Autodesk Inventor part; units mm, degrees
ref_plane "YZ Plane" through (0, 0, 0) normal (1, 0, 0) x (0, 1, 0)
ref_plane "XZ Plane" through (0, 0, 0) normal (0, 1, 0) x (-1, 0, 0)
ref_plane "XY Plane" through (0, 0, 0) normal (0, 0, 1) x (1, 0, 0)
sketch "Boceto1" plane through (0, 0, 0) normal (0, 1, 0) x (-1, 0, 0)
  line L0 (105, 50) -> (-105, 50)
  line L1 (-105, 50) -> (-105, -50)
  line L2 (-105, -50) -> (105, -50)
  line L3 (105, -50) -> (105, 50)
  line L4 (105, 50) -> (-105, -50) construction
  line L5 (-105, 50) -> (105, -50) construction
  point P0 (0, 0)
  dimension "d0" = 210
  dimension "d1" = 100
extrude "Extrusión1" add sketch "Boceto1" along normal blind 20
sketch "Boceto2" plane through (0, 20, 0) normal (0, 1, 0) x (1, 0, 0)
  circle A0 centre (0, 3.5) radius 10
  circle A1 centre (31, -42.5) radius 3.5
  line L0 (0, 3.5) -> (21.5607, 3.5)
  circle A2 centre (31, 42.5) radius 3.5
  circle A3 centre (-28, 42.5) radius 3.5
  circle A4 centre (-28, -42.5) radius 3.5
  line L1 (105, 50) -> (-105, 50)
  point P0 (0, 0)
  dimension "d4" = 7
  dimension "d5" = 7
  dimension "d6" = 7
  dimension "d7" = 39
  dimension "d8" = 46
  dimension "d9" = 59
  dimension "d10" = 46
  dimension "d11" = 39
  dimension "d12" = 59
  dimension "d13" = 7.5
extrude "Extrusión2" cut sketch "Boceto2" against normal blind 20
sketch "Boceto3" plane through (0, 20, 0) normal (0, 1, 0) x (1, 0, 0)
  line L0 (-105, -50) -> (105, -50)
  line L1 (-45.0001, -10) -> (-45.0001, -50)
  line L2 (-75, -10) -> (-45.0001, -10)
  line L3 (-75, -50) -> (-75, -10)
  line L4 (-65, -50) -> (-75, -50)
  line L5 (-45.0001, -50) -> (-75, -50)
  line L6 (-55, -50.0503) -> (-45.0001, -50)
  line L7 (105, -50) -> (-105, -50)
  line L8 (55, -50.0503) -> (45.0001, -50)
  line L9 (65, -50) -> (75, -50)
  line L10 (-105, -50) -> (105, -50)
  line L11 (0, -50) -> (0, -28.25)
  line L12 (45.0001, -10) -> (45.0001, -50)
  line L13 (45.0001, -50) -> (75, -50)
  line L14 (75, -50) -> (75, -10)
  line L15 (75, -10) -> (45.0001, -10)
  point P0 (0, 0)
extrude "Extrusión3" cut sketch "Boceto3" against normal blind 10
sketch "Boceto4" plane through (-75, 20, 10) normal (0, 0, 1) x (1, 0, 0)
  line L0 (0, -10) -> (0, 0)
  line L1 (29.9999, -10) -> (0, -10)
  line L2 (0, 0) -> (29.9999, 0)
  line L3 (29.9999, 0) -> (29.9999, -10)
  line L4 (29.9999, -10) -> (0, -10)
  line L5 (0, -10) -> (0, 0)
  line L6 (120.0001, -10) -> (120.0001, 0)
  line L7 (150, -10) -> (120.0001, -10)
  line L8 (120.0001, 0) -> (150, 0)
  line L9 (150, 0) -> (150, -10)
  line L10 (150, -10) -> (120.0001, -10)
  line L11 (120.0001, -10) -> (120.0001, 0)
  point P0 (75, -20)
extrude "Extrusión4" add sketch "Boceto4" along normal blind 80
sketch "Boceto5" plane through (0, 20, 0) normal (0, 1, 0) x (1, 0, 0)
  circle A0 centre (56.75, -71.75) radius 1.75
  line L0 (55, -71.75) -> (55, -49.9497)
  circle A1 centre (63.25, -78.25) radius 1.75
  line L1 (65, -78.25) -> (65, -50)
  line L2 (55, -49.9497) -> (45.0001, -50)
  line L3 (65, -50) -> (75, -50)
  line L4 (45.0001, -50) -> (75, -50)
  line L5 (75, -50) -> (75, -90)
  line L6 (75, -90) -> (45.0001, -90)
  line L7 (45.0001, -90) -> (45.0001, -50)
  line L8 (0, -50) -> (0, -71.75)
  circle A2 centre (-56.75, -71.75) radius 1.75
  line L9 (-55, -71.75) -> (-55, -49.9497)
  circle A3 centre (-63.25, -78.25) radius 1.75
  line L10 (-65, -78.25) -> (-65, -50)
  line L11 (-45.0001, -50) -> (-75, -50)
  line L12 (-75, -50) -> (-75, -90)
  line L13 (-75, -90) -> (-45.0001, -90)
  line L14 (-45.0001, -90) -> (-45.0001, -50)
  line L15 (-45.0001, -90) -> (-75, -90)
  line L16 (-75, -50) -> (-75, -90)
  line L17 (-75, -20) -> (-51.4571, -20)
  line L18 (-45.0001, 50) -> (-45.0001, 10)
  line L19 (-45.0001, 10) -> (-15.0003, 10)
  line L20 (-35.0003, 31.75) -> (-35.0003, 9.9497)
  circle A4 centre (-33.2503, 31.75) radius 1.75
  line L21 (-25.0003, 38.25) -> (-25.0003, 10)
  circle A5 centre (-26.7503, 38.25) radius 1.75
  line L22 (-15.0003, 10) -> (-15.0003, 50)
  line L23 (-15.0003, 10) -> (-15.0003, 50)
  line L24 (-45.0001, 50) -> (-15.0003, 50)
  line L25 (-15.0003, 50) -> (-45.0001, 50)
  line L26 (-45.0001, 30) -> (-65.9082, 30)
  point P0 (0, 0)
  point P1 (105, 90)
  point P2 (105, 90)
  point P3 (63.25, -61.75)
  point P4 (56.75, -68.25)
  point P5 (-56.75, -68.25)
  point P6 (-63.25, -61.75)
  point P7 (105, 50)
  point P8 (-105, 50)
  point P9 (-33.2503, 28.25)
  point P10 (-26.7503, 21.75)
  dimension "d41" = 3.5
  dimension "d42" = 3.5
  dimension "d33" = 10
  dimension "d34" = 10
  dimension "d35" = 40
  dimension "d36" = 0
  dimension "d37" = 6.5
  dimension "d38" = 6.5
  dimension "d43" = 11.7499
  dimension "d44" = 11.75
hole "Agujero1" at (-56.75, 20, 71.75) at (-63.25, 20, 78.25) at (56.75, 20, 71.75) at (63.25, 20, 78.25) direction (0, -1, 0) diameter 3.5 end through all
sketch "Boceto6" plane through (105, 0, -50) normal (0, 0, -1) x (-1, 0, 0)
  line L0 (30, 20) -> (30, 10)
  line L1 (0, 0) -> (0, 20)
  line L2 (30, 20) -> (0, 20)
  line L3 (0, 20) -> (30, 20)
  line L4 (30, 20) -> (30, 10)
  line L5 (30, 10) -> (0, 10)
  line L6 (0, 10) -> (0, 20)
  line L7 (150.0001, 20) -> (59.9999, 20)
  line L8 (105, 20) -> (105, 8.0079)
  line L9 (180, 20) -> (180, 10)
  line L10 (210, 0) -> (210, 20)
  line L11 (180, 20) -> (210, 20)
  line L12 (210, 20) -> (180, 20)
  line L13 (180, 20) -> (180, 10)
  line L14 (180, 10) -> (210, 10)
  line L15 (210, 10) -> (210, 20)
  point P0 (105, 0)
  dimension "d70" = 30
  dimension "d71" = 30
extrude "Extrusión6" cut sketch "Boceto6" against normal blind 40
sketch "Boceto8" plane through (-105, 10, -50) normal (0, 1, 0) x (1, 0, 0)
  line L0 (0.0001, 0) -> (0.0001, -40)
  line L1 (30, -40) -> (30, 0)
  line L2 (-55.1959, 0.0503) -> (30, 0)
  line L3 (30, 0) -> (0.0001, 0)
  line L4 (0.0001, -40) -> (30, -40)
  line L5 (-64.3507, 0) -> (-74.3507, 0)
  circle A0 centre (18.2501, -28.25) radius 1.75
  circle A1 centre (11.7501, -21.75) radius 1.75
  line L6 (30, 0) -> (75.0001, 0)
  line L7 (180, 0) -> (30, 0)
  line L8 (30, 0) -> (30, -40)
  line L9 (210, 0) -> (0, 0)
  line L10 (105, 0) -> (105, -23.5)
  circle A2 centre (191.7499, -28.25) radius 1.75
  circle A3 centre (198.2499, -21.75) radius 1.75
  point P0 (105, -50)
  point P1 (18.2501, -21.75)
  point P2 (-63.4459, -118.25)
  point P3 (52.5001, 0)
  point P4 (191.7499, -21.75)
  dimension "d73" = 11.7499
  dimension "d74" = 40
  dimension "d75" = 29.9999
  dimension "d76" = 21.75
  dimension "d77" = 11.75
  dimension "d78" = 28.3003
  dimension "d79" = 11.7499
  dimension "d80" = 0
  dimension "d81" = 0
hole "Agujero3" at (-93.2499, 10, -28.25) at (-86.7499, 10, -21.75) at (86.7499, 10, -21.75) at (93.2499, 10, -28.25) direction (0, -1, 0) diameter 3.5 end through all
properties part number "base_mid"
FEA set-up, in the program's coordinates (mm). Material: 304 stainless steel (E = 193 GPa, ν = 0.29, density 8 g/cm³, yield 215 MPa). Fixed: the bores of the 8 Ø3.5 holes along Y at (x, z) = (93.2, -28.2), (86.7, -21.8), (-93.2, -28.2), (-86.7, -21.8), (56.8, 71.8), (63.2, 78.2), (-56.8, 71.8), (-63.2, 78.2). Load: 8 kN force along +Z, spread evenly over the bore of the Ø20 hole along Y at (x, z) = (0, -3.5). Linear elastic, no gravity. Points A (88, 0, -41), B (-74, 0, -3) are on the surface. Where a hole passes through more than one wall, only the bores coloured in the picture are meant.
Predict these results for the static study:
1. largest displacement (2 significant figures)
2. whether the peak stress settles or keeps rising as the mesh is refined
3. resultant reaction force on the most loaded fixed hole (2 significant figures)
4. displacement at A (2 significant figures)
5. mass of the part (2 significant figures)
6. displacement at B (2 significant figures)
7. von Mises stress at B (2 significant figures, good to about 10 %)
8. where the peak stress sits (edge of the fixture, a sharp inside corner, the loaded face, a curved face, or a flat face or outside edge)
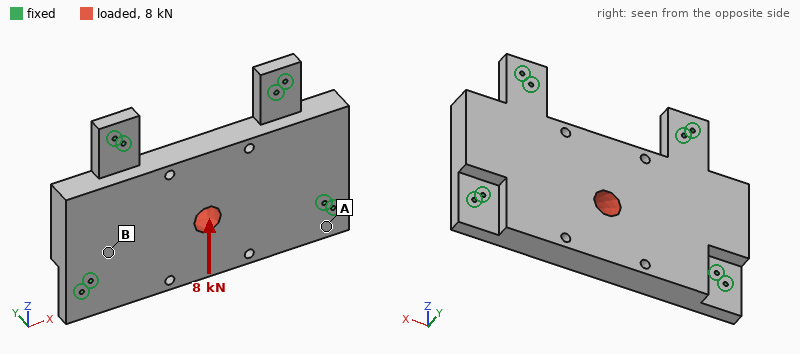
5.0 µm
keeps rising
1.5 kN
0.78 µm
3.3 kg
1.3 µm
4.5 MPa
edge of the fixture
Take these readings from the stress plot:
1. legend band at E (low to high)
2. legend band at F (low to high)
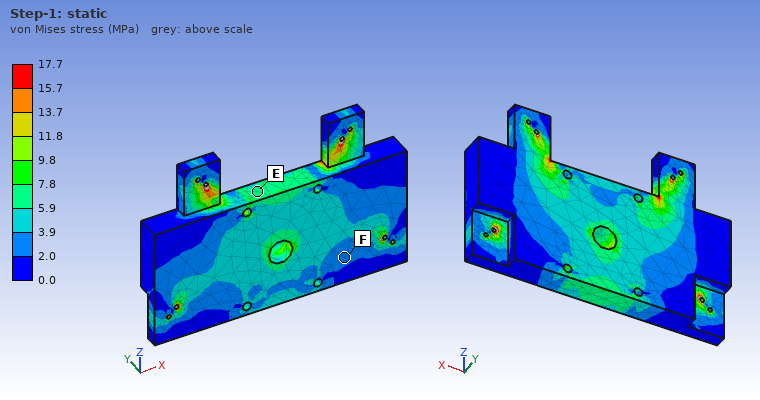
5.9 to 7.8 MPa
2.0 to 3.9 MPa
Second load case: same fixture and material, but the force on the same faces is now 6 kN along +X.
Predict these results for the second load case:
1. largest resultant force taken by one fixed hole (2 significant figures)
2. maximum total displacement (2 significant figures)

1.6 kN
2.1 µm
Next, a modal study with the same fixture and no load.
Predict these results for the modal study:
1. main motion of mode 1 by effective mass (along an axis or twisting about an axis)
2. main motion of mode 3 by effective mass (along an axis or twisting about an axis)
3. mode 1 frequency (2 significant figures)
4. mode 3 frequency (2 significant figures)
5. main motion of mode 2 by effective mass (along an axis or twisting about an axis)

along Y
twisting about Z
2000 Hz
3800 Hz
along Y
